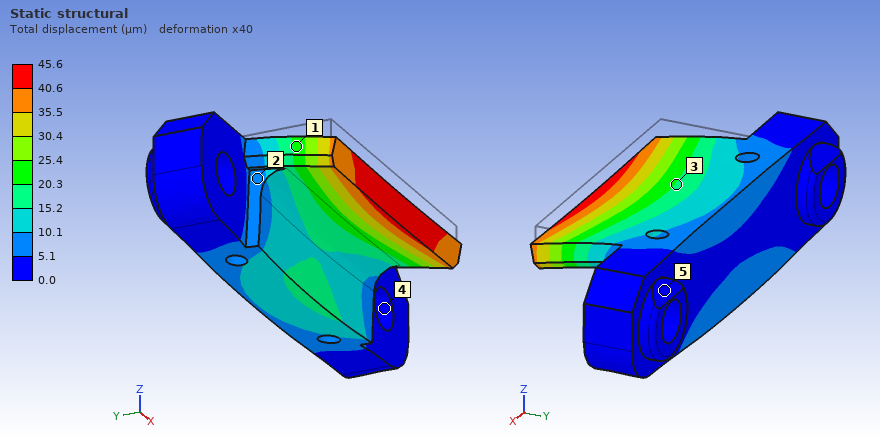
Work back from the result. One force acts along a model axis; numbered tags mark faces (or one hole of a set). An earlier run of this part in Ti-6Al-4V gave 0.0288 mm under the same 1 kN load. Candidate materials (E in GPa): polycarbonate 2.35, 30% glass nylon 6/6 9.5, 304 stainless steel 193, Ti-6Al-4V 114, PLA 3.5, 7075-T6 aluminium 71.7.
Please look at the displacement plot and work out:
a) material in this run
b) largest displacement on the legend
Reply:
7075-T6 aluminium
45.6 µm
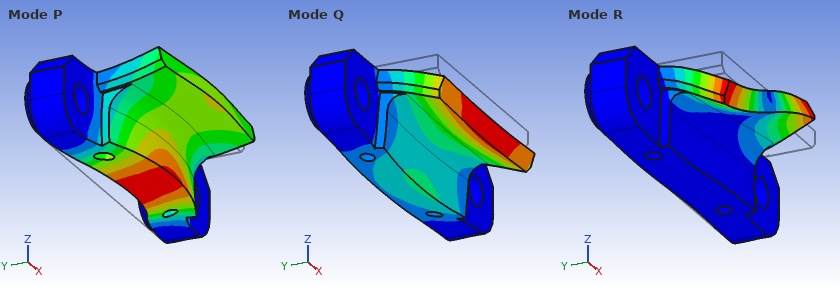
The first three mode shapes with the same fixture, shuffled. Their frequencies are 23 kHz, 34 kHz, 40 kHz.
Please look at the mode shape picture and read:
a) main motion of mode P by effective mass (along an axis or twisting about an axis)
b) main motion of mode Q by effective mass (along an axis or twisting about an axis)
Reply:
along Y
along Z
